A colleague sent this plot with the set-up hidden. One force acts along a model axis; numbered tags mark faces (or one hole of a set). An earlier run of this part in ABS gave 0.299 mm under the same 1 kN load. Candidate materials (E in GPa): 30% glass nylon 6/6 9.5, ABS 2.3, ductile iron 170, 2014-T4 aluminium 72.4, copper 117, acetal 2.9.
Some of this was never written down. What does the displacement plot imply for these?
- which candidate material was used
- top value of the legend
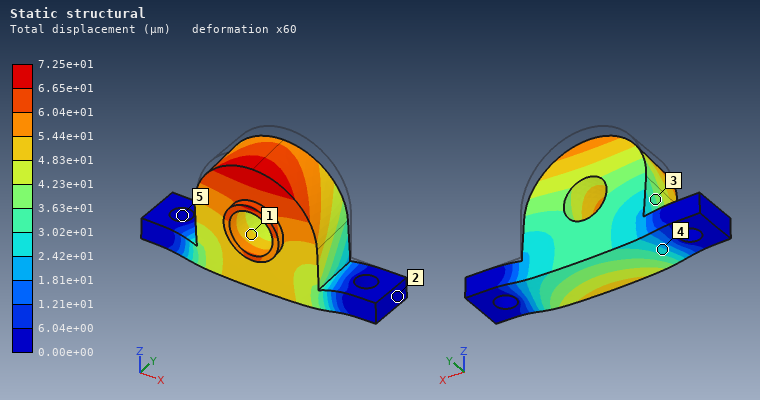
30% glass nylon 6/6
7.25e+01 µm
